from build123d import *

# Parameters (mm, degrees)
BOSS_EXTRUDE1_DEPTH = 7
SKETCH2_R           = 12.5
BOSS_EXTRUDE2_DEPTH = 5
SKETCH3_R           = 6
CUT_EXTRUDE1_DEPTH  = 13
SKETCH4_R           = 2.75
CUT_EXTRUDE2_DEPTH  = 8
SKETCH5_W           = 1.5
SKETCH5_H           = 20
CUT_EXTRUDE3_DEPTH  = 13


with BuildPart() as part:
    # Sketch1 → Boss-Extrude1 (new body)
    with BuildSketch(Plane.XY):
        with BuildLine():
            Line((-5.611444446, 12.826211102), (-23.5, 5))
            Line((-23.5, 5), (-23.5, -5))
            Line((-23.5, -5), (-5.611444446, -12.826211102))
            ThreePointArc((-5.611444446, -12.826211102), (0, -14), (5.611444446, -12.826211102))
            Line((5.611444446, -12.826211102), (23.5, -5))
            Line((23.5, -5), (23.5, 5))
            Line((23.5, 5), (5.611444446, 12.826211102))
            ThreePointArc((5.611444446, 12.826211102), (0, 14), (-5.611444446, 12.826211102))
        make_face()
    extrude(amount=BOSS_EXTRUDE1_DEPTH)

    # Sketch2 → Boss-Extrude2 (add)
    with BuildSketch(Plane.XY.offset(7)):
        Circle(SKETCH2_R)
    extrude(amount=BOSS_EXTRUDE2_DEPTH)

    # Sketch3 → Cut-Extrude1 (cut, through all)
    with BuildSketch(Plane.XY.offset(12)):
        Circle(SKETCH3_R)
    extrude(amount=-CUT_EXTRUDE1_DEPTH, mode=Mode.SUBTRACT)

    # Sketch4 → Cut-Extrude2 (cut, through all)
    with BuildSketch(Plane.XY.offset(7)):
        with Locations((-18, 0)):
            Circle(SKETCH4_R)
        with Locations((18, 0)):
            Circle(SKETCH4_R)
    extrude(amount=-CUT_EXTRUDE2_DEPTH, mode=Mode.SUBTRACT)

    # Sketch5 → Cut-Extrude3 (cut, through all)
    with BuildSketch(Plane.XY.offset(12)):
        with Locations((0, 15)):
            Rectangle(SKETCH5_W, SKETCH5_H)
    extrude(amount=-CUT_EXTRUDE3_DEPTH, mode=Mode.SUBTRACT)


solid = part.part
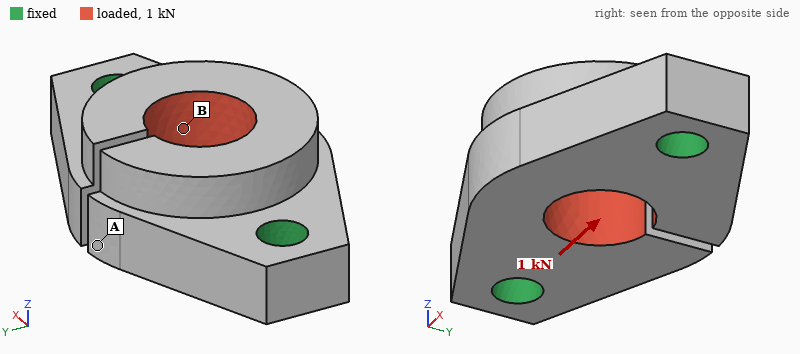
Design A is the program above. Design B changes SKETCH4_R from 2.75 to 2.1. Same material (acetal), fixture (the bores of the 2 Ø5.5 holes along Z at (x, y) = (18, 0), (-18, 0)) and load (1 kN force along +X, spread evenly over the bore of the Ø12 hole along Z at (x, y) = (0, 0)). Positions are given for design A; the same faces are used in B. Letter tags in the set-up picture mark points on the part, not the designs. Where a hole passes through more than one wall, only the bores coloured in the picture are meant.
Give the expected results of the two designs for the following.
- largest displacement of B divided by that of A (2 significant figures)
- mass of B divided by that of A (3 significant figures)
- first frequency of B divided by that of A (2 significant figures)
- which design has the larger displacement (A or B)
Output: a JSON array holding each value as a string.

["1.1", "1.02", "0.92", "B"]
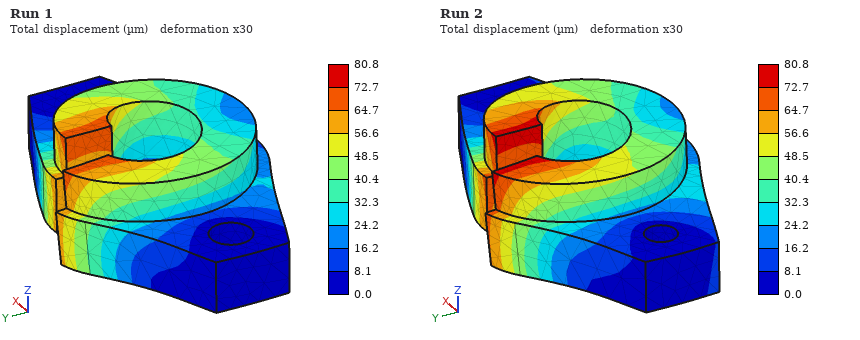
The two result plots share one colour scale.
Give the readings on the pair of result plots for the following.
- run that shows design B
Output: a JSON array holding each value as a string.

["Run 2"]
